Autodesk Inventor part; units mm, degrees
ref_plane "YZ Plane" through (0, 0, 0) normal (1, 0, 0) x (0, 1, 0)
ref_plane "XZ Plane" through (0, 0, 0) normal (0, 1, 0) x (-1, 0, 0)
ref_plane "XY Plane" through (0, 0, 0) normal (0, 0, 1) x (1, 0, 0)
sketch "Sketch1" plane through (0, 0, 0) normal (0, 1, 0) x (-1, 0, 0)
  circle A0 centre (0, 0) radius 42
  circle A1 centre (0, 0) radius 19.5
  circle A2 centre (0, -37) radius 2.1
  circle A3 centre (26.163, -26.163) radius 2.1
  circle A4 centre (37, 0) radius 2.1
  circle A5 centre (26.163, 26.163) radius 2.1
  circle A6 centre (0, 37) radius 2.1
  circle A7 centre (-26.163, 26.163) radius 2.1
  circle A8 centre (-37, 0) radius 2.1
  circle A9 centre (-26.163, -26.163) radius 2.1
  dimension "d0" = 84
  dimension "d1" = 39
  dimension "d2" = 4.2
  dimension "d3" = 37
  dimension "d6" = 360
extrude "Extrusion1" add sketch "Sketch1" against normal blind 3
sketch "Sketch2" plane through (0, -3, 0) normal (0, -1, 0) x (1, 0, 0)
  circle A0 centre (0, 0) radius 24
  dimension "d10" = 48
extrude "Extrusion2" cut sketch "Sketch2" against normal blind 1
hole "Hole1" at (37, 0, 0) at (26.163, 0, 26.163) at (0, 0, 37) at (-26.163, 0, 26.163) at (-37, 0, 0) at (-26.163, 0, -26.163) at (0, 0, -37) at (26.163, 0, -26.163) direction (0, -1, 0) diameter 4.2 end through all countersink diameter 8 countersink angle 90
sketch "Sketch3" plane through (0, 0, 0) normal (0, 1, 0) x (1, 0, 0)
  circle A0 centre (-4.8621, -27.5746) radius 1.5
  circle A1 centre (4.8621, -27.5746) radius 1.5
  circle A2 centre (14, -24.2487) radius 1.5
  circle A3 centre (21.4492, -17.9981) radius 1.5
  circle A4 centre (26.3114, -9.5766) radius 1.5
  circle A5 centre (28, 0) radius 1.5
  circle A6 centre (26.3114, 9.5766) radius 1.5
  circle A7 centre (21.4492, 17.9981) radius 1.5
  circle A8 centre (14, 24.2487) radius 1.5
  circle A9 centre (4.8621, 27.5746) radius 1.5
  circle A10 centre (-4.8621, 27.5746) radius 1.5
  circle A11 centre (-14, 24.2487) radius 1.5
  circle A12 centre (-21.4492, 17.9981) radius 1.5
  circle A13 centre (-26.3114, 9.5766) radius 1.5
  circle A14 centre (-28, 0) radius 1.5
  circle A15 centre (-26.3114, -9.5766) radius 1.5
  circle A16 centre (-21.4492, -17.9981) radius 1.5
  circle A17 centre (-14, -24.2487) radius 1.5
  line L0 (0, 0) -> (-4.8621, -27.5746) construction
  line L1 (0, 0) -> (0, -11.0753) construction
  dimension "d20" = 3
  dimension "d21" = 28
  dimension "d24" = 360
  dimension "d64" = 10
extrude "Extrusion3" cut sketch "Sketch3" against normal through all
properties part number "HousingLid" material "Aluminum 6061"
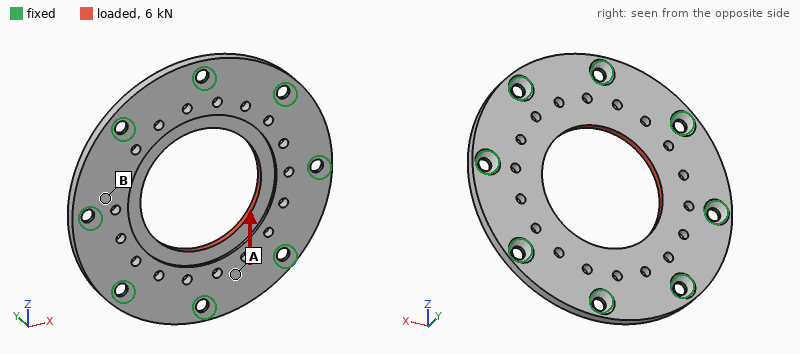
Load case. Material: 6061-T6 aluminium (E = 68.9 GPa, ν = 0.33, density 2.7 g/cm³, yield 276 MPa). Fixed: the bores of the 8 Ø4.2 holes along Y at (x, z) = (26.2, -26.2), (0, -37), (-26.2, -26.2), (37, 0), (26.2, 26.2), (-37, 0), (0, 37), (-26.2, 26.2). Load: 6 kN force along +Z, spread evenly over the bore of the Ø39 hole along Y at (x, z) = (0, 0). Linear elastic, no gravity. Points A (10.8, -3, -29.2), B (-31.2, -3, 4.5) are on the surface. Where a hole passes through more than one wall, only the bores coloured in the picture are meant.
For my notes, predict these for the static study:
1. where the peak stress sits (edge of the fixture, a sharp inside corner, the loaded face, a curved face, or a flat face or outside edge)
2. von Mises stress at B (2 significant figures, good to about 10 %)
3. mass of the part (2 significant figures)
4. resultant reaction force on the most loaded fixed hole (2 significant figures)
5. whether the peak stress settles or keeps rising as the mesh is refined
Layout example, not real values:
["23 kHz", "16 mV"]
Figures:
["edge of the fixture", "19 MPa", "31 g", "1.0 kN", "keeps rising"]
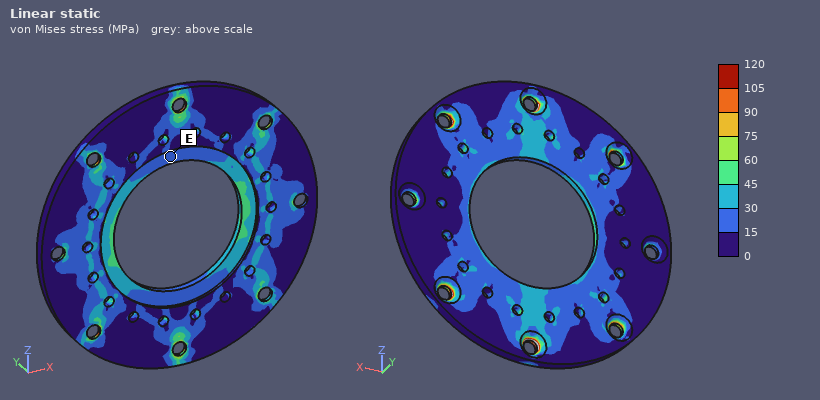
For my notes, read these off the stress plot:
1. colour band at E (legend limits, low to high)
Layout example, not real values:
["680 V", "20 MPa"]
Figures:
["15 to 30 MPa"]
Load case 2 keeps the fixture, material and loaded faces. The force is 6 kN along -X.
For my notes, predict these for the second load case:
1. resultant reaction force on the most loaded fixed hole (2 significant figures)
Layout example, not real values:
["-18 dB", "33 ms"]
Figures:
["1.0 kN"]
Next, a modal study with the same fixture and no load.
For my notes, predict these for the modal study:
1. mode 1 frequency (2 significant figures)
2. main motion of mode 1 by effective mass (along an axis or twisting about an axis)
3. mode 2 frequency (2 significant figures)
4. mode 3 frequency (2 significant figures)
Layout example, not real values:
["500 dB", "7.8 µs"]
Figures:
["7200 Hz", "along Y", "8500 Hz", "8500 Hz"]
